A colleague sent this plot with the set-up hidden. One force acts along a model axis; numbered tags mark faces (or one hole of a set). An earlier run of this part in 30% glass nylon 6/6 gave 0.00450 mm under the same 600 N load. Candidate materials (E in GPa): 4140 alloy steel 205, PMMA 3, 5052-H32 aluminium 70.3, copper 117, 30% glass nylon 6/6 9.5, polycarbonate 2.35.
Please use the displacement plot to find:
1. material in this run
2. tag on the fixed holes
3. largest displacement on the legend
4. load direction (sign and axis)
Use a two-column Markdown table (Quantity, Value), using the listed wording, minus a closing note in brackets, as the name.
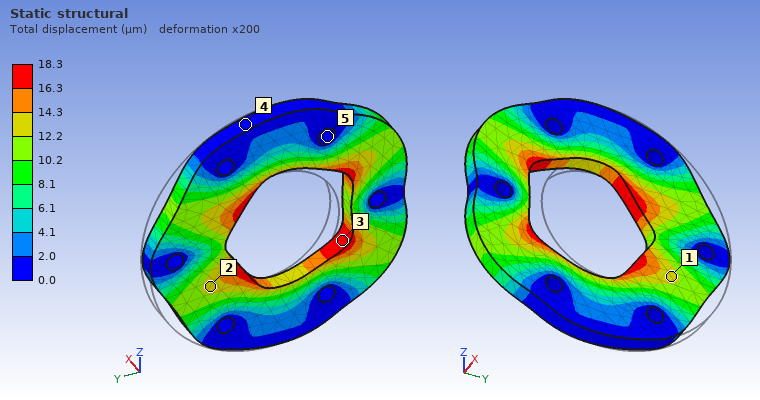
| Quantity | Value |
|---|---|
| material in this run | polycarbonate |
| tag on the fixed holes | 5 |
| largest displacement on the legend | 18.3 µm |
| load direction | -Y |
